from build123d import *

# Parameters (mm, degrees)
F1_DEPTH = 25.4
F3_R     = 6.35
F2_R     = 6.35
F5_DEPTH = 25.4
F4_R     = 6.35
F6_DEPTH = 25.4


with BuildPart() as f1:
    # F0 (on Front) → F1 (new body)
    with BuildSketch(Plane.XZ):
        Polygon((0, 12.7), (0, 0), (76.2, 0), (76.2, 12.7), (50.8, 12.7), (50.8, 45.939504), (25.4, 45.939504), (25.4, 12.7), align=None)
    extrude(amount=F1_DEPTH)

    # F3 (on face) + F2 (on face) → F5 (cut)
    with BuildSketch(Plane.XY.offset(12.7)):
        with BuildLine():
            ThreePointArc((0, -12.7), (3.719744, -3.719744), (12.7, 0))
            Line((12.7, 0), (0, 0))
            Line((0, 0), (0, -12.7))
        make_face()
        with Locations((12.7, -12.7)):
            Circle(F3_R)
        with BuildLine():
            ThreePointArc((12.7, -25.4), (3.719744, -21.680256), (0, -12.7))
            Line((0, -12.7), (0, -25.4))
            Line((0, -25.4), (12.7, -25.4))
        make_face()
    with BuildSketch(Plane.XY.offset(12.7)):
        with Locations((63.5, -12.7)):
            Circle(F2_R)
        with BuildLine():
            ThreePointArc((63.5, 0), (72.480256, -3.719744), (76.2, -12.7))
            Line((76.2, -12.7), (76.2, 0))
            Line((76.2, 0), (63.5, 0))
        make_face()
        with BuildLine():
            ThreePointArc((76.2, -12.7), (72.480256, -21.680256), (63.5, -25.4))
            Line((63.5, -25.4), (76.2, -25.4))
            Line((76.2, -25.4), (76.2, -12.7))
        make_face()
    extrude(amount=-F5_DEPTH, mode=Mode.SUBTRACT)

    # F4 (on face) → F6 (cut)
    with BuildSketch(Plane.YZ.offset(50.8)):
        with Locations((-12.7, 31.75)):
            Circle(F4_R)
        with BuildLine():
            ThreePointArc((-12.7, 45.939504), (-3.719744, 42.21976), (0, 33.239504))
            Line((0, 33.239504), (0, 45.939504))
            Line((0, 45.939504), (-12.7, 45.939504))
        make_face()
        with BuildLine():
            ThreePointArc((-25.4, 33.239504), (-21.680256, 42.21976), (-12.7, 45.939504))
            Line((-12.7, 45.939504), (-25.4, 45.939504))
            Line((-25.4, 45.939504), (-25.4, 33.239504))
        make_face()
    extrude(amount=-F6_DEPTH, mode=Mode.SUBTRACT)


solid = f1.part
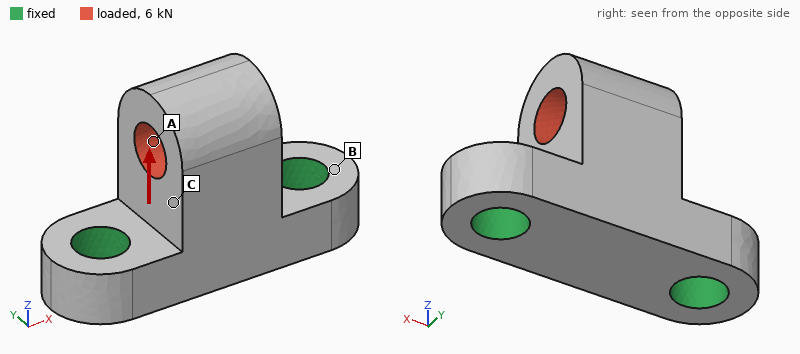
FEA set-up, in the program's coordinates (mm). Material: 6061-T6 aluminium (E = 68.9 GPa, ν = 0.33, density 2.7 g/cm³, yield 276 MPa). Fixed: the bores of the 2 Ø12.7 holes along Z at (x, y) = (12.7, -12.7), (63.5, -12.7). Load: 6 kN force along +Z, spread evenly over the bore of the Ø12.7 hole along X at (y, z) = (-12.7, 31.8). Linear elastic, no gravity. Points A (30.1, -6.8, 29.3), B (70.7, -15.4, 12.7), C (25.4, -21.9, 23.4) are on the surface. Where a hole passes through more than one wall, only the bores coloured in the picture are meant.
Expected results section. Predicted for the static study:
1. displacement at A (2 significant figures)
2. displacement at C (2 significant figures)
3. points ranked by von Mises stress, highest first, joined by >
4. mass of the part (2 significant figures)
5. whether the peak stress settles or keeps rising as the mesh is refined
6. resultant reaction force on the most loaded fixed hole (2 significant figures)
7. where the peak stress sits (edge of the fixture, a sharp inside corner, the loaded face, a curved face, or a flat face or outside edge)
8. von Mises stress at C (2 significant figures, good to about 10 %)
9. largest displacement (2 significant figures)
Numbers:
9.9 µm
9.0 µm
A > C > B
97 g
keeps rising
3.1 kN
edge of the fixture
12 MPa
13 µm
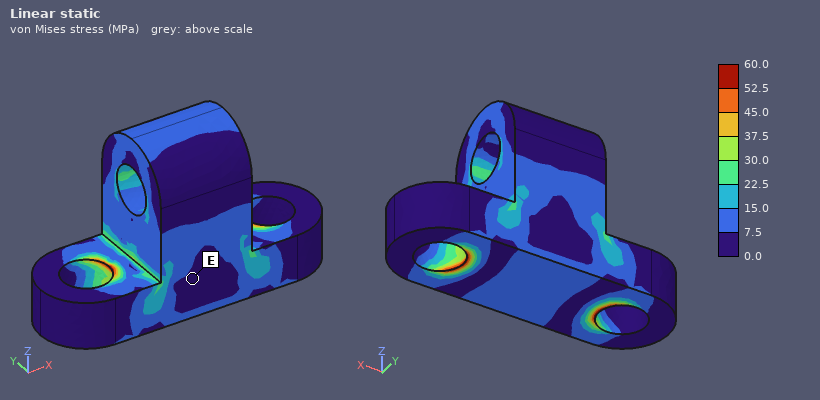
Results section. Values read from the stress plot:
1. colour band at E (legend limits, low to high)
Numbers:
0.0 to 7.5 MPa
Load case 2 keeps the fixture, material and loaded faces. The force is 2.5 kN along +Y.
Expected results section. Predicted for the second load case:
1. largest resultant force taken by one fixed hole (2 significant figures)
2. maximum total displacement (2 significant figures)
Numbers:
1.3 kN
57 µm
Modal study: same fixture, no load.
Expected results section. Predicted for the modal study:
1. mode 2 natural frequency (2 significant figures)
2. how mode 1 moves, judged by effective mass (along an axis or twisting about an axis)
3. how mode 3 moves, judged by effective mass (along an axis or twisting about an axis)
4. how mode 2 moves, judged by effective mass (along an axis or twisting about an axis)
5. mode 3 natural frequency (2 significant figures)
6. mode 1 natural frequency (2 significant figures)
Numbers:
11 kHz
along Y
along Z
along X
17 kHz
6500 Hz
